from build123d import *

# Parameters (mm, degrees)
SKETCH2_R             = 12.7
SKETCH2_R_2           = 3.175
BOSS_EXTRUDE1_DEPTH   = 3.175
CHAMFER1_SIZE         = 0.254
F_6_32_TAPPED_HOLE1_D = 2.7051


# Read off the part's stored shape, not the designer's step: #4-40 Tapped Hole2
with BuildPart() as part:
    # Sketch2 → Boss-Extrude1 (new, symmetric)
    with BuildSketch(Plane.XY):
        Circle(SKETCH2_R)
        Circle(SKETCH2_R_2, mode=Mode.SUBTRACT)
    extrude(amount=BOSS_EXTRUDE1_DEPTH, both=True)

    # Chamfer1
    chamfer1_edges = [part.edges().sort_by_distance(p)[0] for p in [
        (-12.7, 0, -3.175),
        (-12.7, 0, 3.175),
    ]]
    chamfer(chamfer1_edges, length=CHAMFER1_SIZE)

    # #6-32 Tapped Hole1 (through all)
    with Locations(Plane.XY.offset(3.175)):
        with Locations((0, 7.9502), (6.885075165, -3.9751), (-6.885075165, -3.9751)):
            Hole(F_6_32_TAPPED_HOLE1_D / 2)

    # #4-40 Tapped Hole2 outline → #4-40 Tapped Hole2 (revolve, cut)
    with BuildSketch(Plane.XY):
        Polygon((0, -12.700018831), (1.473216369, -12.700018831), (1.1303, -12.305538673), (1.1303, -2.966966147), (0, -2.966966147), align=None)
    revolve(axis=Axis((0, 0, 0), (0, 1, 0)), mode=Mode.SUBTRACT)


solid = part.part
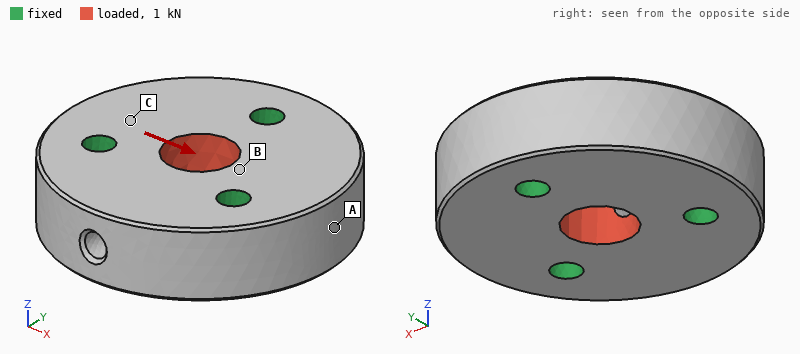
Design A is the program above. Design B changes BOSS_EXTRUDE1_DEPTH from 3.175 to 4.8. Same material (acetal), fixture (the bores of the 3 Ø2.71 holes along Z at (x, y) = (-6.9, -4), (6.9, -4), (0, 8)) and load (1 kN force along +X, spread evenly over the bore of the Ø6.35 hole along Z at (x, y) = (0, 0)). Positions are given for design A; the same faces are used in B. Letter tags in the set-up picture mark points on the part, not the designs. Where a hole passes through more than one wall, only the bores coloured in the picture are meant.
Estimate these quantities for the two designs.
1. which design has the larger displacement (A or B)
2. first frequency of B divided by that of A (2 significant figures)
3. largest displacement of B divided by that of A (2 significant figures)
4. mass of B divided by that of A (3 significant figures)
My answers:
A
1.2
0.67
1.52
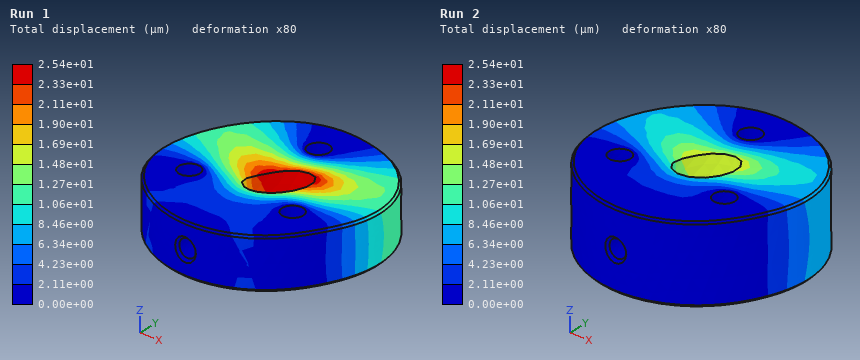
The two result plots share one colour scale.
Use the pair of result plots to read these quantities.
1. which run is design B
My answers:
Run 2
